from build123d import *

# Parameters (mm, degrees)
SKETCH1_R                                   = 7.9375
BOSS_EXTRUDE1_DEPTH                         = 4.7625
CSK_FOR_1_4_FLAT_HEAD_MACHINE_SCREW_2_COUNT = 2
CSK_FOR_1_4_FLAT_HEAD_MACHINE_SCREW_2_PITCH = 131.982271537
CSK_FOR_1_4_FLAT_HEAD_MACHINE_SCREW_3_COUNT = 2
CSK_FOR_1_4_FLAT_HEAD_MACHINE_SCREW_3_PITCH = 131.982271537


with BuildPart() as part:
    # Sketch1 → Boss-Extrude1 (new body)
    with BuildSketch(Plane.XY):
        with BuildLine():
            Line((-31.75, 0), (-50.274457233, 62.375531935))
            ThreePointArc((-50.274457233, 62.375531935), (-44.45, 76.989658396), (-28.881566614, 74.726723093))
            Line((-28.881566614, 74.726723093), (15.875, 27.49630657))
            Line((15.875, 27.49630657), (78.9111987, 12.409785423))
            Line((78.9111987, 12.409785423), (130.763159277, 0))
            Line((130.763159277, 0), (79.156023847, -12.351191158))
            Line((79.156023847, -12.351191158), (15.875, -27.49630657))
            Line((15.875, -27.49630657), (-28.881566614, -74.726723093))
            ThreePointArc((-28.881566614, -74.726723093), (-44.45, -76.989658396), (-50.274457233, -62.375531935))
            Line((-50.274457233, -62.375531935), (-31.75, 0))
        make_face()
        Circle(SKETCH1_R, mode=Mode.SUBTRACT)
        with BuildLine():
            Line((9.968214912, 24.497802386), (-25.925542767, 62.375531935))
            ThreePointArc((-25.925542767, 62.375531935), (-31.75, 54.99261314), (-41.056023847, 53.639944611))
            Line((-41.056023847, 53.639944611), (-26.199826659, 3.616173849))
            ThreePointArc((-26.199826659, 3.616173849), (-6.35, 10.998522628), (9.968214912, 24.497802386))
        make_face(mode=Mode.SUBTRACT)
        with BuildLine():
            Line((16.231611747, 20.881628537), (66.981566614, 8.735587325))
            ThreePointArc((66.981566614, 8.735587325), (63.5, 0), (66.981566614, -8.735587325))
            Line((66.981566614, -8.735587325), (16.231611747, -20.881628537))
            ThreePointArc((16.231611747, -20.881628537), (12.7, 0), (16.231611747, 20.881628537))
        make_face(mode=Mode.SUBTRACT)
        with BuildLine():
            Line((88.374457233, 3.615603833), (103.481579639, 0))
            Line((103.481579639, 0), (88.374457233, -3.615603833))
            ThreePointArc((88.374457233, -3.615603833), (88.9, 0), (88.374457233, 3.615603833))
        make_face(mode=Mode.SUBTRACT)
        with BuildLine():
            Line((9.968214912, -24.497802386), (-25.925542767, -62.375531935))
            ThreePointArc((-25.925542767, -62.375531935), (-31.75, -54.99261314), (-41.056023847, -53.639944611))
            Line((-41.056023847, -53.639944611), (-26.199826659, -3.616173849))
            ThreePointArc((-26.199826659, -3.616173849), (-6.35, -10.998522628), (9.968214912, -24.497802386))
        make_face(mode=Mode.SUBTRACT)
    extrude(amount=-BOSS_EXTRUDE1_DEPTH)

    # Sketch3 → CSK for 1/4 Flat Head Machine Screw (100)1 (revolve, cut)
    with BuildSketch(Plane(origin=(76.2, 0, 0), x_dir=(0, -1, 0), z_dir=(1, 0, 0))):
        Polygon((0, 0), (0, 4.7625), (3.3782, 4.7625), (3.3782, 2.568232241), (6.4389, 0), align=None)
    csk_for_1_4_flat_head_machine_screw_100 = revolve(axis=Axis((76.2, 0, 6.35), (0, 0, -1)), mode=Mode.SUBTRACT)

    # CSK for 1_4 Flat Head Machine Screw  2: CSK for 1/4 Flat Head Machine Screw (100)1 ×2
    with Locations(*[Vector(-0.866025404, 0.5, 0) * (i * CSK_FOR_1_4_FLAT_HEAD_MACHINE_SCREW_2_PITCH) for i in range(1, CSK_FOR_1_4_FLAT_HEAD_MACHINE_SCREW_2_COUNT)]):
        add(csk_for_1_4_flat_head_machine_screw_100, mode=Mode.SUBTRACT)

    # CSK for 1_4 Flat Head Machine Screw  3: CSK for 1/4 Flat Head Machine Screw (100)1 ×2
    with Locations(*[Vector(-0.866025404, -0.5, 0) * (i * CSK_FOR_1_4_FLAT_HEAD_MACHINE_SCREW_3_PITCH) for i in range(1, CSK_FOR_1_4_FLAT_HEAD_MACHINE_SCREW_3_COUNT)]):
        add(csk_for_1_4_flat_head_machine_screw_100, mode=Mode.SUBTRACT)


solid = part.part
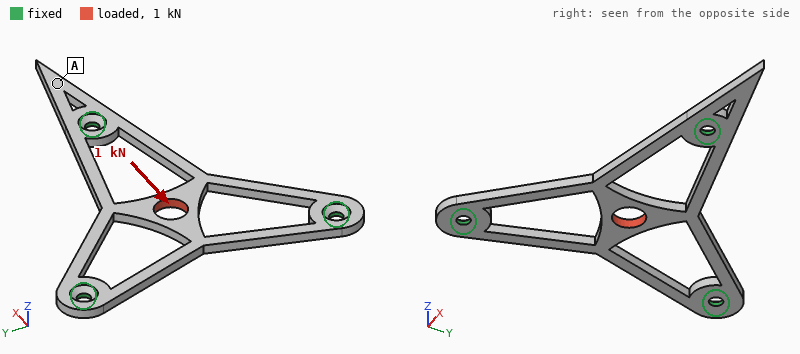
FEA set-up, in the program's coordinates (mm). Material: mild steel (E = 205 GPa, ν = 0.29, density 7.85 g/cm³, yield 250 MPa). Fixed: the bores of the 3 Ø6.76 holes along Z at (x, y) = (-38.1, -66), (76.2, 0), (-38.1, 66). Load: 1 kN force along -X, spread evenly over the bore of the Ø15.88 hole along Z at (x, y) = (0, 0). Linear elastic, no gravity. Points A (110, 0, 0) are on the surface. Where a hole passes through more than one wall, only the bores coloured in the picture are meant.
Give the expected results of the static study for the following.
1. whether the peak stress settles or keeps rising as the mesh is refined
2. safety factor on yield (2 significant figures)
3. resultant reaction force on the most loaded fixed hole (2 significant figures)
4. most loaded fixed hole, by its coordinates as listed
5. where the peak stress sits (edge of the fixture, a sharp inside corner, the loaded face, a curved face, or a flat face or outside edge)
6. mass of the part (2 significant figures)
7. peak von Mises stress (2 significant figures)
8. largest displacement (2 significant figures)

settles
4.1
720 N
(76.2, 0)
a curved face
180 g
61 MPa
17 µm
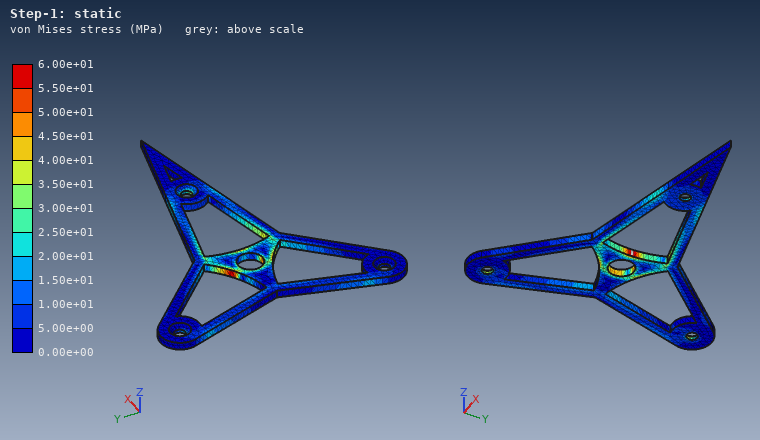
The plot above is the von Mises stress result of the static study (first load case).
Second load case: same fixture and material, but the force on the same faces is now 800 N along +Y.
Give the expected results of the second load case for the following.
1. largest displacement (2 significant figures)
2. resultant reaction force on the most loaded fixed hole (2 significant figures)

13 µm
500 N
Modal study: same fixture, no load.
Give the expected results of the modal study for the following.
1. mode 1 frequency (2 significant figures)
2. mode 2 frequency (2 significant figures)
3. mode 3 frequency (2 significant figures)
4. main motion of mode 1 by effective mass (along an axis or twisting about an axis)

1100 Hz
1900 Hz
2000 Hz
along Z
